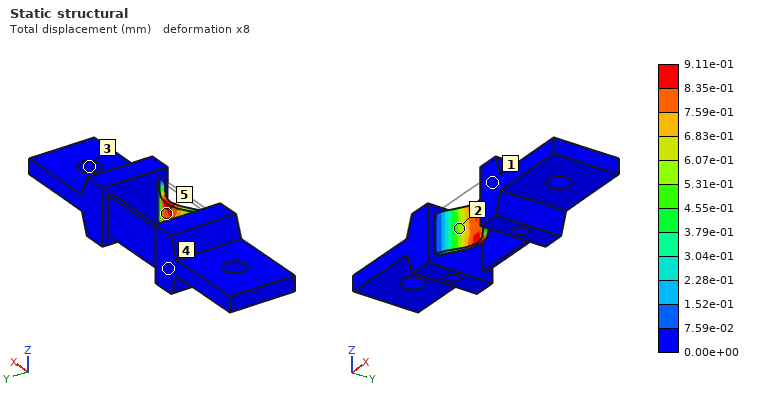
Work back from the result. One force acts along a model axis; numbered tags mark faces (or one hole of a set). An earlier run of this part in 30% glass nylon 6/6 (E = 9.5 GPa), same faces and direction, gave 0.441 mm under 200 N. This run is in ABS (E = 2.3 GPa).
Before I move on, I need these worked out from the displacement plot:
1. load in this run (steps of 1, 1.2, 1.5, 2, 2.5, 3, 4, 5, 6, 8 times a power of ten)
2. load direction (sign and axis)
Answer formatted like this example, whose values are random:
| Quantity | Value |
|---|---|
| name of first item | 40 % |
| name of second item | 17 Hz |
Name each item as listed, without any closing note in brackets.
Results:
| Quantity | Value |
|---|---|
| load in this run | 100 N |
| load direction | +Y |
